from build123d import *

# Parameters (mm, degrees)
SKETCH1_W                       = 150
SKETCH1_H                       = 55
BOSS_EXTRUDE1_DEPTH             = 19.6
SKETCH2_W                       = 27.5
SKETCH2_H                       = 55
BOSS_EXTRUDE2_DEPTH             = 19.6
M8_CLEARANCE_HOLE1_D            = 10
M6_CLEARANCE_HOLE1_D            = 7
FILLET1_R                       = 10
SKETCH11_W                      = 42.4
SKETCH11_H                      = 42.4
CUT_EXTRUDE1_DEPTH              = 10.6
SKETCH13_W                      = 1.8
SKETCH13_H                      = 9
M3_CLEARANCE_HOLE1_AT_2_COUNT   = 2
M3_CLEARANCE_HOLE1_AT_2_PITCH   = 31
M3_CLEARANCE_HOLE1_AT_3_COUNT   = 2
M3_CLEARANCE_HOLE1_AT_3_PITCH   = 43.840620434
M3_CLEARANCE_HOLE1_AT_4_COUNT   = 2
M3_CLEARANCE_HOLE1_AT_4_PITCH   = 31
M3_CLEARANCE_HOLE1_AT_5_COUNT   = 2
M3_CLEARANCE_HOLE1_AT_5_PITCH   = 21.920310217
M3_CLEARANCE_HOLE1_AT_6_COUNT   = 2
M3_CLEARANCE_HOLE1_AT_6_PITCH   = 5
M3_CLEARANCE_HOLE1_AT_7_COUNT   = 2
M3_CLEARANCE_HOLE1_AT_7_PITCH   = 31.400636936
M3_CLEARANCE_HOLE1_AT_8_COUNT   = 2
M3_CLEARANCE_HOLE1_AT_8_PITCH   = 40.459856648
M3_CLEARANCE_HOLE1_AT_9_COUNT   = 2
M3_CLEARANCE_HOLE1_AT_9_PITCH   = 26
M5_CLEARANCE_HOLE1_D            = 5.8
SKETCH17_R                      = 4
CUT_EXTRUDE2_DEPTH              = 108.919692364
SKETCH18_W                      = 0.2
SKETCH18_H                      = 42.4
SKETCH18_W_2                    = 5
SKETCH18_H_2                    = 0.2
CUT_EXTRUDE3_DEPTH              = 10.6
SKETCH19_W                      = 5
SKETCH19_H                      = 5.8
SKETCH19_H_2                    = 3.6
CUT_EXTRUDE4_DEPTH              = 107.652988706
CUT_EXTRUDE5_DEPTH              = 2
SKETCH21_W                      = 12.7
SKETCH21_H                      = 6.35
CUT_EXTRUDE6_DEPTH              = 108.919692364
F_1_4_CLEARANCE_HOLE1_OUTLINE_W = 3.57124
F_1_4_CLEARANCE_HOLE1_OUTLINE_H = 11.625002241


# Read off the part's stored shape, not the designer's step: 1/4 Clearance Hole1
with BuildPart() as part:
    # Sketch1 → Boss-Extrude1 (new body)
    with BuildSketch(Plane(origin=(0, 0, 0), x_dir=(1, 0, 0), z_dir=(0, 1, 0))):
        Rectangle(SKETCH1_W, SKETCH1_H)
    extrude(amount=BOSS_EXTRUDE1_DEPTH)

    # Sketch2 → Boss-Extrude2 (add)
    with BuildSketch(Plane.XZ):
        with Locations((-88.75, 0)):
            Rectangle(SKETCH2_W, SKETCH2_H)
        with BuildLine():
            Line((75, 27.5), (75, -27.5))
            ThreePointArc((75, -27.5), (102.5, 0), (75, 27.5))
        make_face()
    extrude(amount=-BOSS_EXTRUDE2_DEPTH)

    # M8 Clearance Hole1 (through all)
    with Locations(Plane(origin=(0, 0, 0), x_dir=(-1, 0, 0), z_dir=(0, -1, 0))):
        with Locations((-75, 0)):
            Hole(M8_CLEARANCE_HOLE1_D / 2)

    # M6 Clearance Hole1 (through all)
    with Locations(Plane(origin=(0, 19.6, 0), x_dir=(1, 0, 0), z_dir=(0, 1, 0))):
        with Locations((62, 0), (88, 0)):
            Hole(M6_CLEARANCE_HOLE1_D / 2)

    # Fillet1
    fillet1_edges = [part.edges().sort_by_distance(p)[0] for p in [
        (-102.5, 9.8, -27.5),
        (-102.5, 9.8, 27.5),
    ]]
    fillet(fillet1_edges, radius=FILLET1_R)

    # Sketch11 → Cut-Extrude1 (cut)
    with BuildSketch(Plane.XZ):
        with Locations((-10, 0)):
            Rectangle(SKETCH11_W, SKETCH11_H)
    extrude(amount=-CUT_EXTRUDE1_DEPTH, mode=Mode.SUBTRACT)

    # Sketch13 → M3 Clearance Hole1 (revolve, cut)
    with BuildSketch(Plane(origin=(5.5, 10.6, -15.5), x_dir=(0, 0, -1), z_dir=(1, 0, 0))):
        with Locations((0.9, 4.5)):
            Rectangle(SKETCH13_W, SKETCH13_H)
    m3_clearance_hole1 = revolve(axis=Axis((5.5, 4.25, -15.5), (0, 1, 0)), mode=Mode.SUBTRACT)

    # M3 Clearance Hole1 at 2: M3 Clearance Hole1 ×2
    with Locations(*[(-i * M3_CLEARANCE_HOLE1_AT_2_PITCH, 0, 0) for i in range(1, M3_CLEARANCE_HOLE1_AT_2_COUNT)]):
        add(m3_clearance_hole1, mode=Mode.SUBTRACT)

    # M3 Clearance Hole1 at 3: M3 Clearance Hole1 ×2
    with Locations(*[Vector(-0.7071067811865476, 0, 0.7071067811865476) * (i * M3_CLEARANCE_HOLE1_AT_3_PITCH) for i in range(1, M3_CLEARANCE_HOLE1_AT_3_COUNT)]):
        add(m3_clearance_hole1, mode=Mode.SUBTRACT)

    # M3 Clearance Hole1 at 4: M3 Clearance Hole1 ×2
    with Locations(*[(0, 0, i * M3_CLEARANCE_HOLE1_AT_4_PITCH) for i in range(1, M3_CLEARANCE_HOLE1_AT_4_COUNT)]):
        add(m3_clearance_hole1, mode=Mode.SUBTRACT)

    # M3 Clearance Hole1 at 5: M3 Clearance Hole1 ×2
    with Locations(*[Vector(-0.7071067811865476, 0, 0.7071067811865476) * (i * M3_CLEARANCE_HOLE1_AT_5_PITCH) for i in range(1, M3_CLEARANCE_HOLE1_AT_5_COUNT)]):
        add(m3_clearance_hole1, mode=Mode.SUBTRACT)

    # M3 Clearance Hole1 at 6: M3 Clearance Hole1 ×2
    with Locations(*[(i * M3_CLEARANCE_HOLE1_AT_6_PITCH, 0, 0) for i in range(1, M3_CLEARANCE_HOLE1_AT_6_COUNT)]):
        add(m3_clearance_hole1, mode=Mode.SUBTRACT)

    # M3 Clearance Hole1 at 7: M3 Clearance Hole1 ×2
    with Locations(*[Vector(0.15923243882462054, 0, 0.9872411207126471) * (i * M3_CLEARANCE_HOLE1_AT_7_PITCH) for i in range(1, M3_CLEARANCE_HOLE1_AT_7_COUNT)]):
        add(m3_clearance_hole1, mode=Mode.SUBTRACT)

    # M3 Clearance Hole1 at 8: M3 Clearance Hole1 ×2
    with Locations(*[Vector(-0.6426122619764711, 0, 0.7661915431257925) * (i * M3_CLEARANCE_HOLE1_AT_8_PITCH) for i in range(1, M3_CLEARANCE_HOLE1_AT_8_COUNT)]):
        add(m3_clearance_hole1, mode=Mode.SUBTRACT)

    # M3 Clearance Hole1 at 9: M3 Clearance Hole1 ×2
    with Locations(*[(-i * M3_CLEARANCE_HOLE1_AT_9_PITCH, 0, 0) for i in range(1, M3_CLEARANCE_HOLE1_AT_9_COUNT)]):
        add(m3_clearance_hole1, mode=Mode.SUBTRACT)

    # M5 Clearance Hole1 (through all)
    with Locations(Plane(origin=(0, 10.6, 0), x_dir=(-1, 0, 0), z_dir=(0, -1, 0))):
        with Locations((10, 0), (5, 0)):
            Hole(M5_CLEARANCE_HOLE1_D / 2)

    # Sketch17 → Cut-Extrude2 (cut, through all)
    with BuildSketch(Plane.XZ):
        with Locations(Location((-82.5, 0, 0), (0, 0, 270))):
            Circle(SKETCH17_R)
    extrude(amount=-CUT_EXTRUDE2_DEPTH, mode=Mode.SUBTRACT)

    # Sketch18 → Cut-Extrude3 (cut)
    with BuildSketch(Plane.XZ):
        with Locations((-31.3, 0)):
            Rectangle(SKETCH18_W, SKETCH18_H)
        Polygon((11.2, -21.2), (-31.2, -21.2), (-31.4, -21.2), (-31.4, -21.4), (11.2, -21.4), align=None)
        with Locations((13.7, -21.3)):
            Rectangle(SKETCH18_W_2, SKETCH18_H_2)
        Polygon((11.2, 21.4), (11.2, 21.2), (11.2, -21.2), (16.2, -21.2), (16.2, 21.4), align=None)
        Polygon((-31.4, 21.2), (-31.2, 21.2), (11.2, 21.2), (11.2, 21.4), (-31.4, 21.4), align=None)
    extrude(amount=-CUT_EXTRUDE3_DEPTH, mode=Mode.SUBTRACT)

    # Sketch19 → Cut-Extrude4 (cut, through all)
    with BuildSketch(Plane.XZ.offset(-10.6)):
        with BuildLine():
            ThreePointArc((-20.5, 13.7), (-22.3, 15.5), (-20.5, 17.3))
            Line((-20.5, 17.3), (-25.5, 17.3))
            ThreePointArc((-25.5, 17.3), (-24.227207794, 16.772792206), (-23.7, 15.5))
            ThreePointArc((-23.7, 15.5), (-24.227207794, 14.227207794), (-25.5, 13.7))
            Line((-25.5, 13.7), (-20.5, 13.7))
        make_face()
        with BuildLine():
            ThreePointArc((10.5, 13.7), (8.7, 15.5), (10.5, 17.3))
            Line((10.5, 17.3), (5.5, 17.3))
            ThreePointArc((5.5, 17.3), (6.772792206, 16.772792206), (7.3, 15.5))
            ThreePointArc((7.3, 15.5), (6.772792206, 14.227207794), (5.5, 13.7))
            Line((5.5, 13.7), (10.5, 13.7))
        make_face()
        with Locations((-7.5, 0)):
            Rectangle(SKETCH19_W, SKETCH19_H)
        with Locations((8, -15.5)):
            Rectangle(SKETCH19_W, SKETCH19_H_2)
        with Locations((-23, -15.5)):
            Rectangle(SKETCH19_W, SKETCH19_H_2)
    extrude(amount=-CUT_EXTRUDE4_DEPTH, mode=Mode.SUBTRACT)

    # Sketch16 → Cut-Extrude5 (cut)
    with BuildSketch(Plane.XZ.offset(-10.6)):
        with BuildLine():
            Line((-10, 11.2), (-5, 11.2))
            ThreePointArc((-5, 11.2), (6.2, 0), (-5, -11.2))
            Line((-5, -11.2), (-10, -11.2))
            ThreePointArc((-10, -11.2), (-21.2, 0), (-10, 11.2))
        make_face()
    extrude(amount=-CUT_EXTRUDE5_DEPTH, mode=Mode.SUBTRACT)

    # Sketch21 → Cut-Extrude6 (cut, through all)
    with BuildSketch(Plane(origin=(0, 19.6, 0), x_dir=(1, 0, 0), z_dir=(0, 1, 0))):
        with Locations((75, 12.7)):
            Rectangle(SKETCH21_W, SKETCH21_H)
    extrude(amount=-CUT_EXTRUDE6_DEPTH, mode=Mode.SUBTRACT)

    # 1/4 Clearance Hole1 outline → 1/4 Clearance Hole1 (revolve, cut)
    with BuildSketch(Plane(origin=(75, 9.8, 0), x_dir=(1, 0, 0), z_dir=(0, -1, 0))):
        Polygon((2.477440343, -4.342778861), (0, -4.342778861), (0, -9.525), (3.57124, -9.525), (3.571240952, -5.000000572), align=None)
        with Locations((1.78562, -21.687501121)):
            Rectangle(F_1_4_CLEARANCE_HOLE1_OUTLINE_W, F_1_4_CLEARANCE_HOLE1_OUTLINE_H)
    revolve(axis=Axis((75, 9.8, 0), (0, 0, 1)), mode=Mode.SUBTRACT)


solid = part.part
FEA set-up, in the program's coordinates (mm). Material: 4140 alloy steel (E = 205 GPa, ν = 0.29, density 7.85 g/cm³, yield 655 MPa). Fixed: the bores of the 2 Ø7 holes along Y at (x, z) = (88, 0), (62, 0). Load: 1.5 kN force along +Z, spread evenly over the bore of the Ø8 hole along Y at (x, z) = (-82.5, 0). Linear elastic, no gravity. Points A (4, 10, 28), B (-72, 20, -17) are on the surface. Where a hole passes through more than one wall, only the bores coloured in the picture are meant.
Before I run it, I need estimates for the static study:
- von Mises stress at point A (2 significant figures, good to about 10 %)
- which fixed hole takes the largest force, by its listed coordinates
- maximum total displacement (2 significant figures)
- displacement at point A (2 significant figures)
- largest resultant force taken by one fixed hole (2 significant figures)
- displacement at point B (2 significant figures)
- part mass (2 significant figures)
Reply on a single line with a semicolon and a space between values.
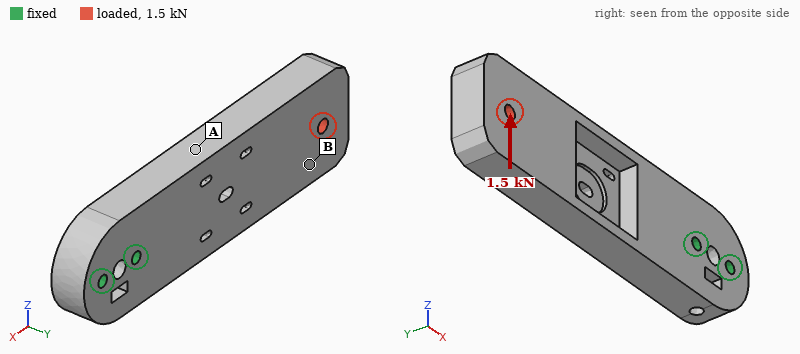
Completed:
20 MPa; (62, 0); 82 µm; 23 µm; 6.9 kN; 59 µm; 1.4 kg
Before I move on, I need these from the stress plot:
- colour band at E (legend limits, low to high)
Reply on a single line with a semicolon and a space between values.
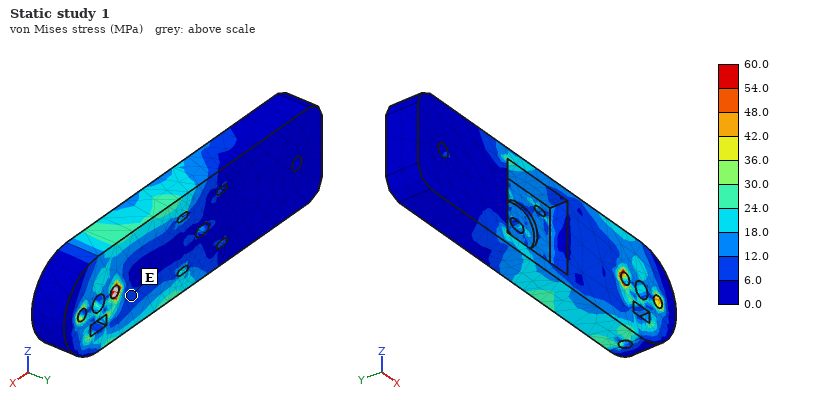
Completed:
6.0 to 12.0 MPa
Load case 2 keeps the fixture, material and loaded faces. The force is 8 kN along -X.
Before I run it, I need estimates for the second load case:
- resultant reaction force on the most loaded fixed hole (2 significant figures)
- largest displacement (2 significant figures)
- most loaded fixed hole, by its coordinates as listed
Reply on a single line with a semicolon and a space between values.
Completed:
6.2 kN; 57 µm; (62, 0)
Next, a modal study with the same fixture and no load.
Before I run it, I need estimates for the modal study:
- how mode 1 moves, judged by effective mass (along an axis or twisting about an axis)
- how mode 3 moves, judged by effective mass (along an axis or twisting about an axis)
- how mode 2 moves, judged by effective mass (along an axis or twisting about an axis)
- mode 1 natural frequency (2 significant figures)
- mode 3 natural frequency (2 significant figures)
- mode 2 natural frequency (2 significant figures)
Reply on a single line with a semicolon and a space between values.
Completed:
along Y; twisting about X; along Z; 480 Hz; 2000 Hz; 1000 Hz
